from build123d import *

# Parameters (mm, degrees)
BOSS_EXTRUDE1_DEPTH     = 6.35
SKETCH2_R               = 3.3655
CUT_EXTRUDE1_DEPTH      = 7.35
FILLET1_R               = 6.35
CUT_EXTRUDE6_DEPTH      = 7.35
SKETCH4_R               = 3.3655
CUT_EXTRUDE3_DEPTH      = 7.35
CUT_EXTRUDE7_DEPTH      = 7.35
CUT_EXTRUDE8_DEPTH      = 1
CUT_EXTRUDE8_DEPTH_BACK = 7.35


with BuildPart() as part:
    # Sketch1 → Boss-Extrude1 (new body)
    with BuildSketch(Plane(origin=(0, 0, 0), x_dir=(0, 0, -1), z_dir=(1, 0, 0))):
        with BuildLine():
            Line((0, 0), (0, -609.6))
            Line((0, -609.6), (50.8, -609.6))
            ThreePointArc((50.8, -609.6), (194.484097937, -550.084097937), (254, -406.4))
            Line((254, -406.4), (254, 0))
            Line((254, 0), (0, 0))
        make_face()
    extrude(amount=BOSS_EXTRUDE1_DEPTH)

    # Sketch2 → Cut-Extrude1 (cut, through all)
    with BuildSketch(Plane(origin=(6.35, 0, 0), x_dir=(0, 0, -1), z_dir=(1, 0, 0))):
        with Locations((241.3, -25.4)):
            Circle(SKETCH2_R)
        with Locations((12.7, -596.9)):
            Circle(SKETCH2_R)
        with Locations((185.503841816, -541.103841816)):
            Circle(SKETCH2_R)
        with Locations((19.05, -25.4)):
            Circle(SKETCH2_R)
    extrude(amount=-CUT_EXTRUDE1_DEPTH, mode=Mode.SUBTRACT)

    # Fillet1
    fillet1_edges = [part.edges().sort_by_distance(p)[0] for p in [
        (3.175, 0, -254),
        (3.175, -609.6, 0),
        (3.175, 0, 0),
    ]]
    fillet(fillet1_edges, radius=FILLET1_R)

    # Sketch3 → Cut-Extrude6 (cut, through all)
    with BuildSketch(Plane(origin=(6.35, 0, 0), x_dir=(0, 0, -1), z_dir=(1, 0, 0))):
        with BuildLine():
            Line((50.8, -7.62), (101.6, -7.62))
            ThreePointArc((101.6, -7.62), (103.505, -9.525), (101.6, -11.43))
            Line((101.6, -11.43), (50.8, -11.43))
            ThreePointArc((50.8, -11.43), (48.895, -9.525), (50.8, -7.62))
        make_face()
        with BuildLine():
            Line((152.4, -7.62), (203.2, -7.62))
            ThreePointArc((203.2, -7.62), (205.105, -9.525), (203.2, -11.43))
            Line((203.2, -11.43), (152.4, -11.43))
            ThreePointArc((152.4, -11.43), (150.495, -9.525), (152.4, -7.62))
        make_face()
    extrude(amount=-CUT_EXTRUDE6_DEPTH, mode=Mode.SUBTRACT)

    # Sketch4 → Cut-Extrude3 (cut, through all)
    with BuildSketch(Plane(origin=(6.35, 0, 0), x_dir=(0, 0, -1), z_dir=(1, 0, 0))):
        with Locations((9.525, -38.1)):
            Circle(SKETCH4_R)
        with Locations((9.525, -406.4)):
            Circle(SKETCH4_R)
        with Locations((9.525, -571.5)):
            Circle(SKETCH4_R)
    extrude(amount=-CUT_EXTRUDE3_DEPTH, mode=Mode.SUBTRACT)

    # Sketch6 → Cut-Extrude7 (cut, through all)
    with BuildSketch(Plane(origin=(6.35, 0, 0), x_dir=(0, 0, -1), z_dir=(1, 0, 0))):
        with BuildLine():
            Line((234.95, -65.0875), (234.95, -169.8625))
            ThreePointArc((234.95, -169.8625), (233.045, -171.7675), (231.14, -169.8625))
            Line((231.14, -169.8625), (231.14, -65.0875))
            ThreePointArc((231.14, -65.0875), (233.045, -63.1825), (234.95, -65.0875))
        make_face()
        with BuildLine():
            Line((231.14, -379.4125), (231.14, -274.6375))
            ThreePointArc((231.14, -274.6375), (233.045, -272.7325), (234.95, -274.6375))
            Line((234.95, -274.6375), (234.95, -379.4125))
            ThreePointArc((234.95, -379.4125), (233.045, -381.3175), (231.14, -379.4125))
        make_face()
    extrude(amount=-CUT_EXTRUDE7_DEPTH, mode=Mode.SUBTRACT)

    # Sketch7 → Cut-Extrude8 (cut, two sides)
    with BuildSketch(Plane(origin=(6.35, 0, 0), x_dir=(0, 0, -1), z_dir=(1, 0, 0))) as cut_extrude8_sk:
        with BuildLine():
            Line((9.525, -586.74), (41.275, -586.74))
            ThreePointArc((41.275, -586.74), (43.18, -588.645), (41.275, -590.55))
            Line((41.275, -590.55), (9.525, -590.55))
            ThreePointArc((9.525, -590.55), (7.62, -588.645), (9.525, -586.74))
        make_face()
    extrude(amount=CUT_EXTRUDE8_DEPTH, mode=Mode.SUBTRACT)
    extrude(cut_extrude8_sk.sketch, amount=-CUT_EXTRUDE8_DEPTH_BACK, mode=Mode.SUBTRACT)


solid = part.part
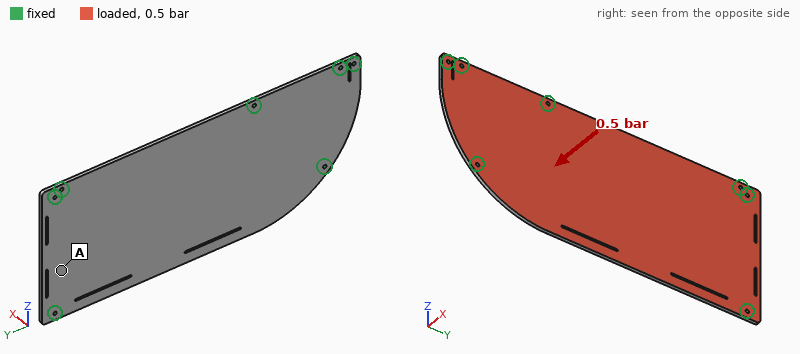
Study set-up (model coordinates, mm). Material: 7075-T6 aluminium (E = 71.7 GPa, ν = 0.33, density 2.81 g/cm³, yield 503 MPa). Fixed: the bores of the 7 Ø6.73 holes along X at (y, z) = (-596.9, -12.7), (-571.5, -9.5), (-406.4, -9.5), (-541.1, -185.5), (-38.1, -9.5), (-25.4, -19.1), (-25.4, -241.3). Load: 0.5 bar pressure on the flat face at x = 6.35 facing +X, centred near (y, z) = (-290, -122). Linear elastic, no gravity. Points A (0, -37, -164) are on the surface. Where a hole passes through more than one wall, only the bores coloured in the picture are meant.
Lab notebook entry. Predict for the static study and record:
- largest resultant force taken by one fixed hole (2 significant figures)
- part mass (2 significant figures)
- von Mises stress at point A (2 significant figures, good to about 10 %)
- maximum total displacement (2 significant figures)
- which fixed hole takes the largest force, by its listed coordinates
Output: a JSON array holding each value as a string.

["2.4 kN", "2.6 kg", "34 MPa", "7.0 mm", "(-406.4, -9.5)"]
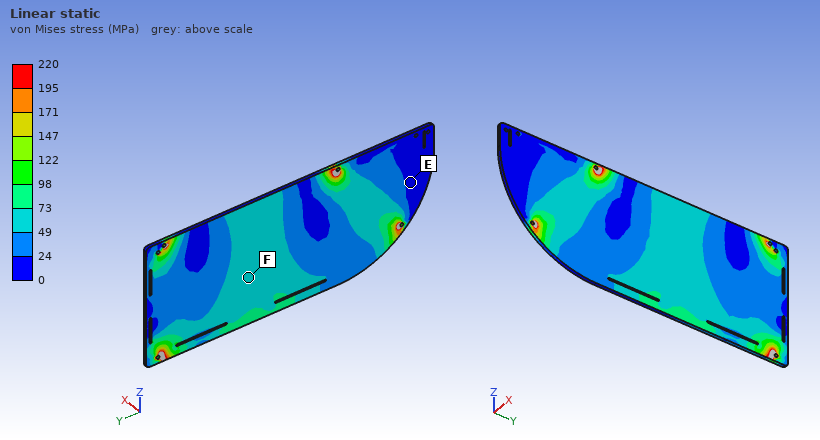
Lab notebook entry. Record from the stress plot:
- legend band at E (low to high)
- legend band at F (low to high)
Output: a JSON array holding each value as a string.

["0 to 24 MPa", "49 to 73 MPa"]
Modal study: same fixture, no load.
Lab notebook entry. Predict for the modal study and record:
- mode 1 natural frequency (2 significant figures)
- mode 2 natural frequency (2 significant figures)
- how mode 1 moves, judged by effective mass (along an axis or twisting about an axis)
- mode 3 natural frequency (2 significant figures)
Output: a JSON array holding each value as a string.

["130 Hz", "260 Hz", "along X", "360 Hz"]
